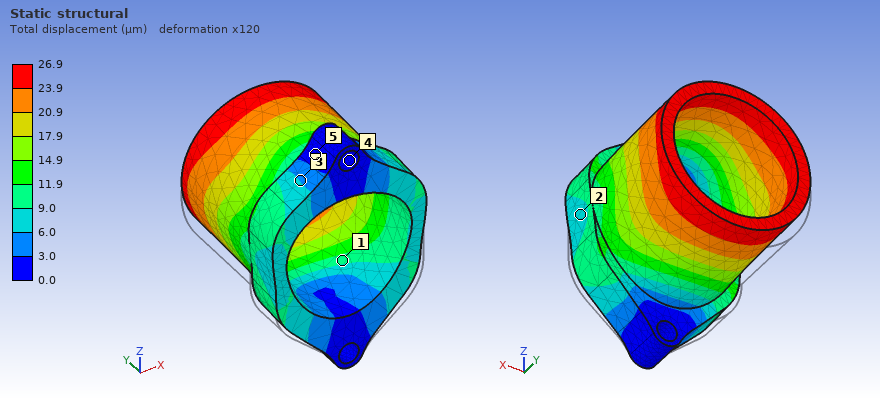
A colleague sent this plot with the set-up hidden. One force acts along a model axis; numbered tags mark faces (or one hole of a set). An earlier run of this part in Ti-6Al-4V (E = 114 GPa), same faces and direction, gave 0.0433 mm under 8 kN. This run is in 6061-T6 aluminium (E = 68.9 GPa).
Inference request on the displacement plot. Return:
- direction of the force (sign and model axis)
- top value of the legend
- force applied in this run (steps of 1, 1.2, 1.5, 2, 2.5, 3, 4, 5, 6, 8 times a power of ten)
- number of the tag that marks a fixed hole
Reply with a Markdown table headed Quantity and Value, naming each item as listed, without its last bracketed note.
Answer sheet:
| Quantity | Value |
|---|---|
| direction of the force | +Z |
| top value of the legend | 26.9 µm |
| force applied in this run | 3 kN |
| number of the tag that marks a fixed hole | 4 |
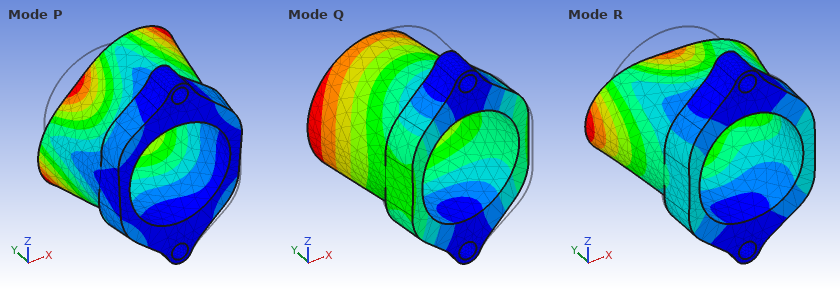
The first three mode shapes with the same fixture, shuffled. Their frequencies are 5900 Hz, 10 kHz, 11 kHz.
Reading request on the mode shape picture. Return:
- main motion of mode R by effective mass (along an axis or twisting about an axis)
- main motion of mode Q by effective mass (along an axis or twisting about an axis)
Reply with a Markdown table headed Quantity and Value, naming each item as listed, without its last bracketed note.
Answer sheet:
| Quantity | Value |
|---|---|
| main motion of mode R by effective mass | along Y |
| main motion of mode Q by effective mass | along X |
